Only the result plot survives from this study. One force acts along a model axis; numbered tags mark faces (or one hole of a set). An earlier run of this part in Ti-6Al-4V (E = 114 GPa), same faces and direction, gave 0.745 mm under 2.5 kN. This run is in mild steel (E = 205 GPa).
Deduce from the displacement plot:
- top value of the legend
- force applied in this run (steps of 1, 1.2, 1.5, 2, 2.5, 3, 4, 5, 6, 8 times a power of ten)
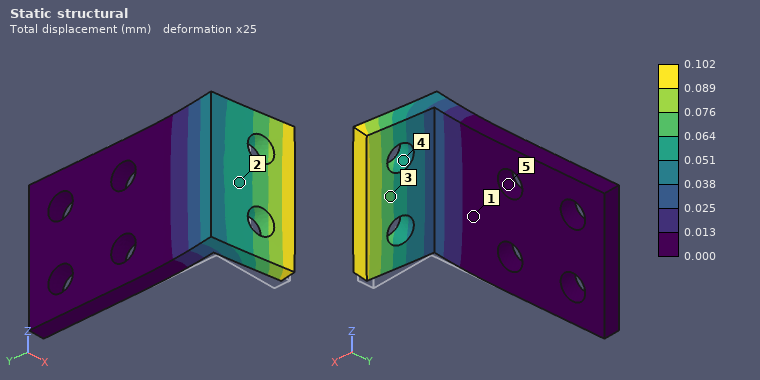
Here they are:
0.102 mm
600 N
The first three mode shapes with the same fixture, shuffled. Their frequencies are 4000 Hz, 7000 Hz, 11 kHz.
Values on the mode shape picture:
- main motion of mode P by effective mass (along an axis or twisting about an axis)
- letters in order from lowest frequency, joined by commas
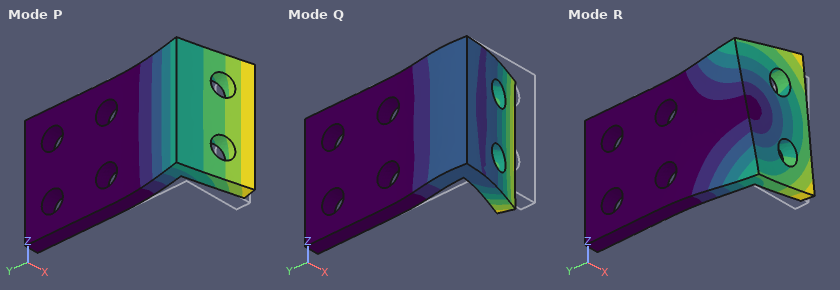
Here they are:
along X
P, R, Q
